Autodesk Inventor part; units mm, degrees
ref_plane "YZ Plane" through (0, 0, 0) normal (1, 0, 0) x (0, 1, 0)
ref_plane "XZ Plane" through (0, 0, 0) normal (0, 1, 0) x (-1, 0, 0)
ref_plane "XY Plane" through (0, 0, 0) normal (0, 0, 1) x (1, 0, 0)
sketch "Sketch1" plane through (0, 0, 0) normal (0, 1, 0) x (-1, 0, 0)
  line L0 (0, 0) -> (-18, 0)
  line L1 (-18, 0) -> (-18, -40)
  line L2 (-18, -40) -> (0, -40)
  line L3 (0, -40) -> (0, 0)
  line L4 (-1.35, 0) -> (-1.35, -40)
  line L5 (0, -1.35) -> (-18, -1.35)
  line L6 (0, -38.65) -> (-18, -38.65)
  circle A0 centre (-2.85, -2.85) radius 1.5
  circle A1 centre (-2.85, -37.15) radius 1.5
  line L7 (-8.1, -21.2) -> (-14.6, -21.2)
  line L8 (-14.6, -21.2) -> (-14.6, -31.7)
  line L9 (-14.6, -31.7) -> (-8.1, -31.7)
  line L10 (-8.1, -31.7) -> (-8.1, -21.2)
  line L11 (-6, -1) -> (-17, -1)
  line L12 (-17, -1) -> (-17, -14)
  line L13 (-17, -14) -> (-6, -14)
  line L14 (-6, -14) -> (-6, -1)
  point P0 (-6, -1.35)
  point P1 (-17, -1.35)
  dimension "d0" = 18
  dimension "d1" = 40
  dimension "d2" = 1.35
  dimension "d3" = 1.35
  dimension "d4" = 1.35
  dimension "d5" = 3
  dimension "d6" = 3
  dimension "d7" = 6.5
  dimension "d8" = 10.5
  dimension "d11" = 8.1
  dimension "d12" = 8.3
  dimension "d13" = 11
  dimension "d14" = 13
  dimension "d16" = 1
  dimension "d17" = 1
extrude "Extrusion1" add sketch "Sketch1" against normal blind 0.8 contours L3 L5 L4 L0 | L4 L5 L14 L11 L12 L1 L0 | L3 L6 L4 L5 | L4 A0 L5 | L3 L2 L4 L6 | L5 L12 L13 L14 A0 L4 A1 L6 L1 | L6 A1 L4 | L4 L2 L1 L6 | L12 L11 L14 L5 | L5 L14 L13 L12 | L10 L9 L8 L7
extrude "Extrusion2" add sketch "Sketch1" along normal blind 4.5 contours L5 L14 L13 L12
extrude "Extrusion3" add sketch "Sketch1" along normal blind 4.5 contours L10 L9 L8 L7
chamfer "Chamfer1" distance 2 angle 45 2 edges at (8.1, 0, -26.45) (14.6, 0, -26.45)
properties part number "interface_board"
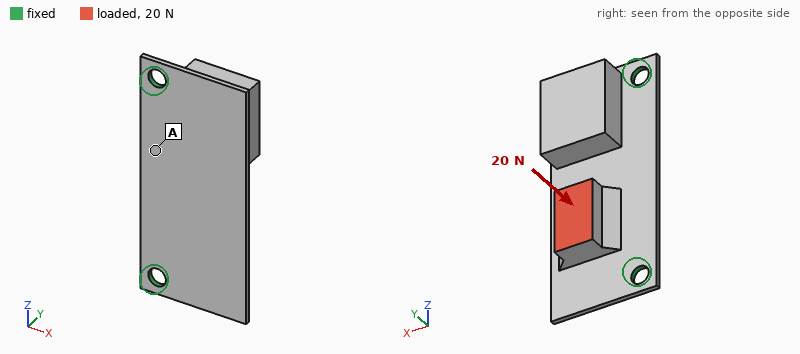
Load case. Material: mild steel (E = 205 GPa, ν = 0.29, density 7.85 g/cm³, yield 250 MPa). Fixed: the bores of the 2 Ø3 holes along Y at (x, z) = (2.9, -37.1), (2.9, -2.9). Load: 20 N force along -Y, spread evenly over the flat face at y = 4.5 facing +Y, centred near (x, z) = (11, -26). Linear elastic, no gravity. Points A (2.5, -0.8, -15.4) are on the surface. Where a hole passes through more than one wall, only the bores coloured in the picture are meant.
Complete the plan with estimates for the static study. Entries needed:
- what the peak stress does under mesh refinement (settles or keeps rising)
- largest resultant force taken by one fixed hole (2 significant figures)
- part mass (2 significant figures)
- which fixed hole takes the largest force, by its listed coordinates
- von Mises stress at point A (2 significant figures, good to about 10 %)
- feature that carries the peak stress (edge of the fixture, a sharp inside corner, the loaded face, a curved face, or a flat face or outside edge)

keeps rising
13 N
12 g
(2.9, -37.1)
14 MPa
edge of the fixture
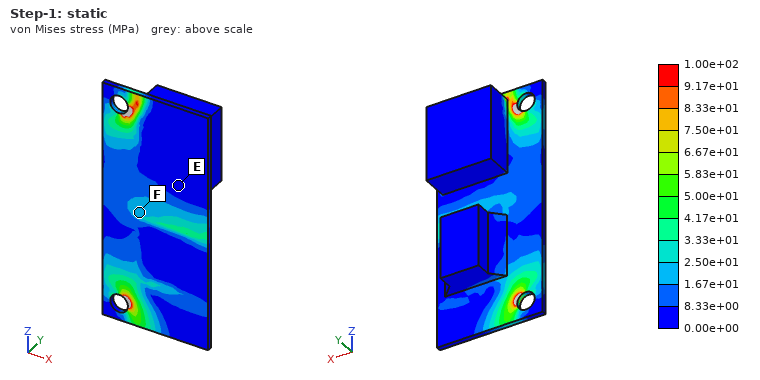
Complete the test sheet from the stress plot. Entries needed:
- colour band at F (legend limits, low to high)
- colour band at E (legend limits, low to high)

1.67e+01 to 2.50e+01 MPa
0.00e+00 to 8.33e+00 MPa
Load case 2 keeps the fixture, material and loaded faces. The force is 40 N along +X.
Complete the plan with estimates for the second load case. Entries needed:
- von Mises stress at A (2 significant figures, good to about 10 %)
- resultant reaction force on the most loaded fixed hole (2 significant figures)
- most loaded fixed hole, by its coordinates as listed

16 MPa
30 N
(2.9, -37.1)
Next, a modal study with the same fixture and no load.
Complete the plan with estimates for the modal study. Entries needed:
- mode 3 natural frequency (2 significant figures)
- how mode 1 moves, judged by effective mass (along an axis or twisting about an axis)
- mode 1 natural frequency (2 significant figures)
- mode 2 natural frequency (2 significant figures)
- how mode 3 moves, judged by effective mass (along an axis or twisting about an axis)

4400 Hz
along Y
1300 Hz
3800 Hz
twisting about X
